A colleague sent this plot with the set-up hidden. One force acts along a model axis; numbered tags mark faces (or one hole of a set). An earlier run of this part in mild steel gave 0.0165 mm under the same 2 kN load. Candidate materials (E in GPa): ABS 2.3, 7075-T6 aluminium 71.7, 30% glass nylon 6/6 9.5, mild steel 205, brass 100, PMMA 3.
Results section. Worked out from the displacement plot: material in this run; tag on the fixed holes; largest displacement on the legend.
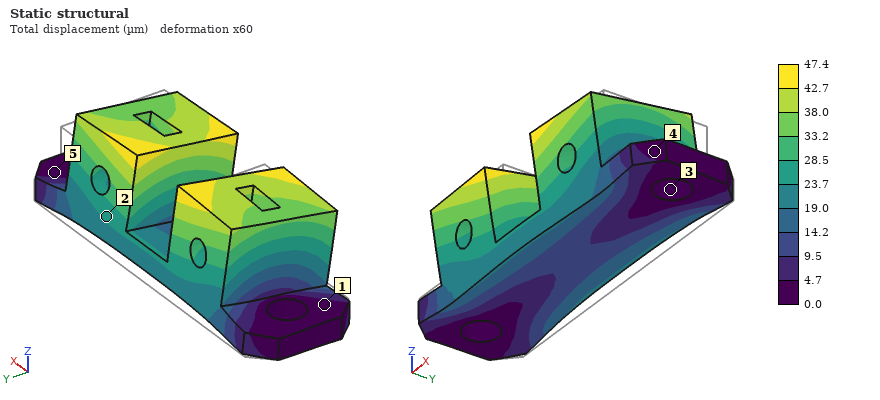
7075-T6 aluminium
3
47.4 µm
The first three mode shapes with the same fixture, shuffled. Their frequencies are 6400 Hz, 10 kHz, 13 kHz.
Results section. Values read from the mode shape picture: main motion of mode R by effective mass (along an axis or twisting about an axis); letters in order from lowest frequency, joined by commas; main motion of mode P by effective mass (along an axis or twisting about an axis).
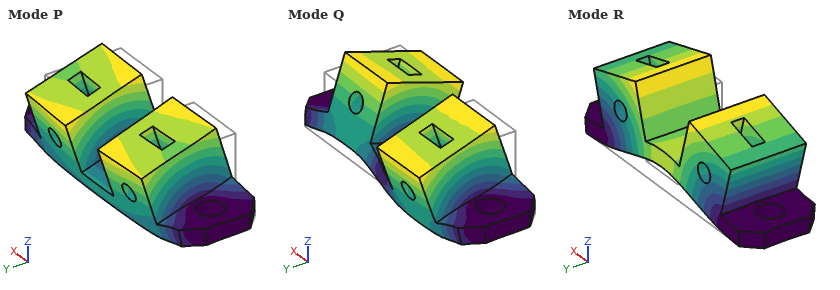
along Z
R, P, Q
along Y
